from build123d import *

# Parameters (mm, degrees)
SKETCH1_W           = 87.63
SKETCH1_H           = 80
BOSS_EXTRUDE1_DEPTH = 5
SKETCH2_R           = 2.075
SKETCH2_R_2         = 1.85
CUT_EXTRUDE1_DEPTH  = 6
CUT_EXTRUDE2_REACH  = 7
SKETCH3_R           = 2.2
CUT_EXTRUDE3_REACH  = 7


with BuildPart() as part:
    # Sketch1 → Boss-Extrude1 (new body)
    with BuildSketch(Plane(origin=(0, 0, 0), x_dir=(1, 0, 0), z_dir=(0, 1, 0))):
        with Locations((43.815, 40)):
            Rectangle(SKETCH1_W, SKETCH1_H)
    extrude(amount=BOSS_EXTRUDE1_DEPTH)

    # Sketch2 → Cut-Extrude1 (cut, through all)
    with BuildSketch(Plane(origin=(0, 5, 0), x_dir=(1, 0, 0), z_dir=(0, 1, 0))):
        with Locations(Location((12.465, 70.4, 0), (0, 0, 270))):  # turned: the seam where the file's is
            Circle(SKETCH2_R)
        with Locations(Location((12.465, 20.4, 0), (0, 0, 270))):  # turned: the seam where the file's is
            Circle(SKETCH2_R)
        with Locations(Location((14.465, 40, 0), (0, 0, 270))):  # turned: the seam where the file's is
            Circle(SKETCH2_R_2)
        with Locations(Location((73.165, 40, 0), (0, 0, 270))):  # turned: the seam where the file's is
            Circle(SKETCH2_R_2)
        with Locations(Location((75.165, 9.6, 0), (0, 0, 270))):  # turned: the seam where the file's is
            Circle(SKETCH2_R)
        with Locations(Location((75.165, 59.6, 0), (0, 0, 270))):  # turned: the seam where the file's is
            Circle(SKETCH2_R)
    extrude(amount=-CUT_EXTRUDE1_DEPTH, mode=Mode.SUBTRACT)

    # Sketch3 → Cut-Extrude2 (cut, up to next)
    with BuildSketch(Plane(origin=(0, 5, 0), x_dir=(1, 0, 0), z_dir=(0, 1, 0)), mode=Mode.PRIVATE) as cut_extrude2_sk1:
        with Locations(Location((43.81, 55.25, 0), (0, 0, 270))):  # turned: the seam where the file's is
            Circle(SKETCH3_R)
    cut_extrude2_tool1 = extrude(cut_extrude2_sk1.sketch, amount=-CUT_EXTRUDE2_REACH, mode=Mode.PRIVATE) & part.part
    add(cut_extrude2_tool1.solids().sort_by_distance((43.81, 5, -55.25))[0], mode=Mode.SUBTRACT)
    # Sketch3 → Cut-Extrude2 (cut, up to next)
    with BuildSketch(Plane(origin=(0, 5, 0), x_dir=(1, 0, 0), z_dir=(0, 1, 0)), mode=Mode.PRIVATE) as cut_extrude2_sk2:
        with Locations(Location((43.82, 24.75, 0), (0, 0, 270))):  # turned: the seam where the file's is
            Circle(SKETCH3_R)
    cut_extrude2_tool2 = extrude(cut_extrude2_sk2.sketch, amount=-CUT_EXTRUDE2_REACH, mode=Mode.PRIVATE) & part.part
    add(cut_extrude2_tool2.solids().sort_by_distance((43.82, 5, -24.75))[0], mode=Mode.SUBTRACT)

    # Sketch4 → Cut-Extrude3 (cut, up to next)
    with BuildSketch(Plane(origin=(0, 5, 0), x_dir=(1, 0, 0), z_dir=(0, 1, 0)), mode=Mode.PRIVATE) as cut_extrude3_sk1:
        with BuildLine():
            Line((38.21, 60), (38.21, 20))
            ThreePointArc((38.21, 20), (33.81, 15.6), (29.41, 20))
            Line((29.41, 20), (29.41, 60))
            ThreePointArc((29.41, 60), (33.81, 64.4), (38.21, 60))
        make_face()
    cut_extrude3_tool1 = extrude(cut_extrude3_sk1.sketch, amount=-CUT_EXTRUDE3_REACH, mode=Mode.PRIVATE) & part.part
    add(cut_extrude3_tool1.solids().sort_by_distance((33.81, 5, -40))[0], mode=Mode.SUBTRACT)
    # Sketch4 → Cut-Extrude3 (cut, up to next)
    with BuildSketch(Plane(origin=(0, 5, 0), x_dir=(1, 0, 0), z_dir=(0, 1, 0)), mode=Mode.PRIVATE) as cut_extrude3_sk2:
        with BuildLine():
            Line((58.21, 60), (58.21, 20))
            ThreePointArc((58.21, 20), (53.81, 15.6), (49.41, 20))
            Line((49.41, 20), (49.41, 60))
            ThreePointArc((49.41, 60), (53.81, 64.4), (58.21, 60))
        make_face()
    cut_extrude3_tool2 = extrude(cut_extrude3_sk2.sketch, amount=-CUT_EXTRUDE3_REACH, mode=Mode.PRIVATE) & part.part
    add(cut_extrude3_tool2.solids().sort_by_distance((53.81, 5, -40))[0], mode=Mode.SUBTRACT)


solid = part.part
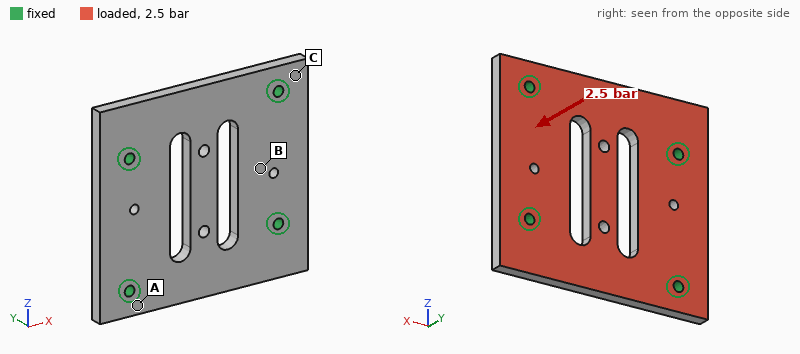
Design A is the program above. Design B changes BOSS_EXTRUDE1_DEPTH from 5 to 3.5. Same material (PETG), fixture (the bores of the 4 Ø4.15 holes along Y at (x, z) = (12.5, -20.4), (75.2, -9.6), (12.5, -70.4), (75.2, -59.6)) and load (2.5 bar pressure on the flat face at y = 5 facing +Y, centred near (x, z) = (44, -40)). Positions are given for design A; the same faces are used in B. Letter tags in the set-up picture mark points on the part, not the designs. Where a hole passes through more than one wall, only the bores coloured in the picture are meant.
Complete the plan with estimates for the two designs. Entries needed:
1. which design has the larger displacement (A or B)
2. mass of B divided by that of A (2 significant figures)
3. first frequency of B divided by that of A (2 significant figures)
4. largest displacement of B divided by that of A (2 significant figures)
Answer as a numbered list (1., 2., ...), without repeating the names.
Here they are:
1. B
2. 0.70
3. 0.74
4. 2.6
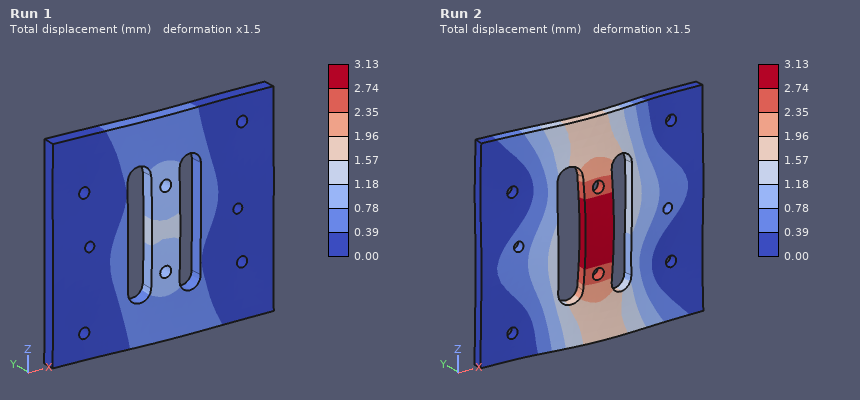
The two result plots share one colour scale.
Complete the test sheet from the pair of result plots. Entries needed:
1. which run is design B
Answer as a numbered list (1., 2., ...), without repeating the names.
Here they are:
1. Run 2
